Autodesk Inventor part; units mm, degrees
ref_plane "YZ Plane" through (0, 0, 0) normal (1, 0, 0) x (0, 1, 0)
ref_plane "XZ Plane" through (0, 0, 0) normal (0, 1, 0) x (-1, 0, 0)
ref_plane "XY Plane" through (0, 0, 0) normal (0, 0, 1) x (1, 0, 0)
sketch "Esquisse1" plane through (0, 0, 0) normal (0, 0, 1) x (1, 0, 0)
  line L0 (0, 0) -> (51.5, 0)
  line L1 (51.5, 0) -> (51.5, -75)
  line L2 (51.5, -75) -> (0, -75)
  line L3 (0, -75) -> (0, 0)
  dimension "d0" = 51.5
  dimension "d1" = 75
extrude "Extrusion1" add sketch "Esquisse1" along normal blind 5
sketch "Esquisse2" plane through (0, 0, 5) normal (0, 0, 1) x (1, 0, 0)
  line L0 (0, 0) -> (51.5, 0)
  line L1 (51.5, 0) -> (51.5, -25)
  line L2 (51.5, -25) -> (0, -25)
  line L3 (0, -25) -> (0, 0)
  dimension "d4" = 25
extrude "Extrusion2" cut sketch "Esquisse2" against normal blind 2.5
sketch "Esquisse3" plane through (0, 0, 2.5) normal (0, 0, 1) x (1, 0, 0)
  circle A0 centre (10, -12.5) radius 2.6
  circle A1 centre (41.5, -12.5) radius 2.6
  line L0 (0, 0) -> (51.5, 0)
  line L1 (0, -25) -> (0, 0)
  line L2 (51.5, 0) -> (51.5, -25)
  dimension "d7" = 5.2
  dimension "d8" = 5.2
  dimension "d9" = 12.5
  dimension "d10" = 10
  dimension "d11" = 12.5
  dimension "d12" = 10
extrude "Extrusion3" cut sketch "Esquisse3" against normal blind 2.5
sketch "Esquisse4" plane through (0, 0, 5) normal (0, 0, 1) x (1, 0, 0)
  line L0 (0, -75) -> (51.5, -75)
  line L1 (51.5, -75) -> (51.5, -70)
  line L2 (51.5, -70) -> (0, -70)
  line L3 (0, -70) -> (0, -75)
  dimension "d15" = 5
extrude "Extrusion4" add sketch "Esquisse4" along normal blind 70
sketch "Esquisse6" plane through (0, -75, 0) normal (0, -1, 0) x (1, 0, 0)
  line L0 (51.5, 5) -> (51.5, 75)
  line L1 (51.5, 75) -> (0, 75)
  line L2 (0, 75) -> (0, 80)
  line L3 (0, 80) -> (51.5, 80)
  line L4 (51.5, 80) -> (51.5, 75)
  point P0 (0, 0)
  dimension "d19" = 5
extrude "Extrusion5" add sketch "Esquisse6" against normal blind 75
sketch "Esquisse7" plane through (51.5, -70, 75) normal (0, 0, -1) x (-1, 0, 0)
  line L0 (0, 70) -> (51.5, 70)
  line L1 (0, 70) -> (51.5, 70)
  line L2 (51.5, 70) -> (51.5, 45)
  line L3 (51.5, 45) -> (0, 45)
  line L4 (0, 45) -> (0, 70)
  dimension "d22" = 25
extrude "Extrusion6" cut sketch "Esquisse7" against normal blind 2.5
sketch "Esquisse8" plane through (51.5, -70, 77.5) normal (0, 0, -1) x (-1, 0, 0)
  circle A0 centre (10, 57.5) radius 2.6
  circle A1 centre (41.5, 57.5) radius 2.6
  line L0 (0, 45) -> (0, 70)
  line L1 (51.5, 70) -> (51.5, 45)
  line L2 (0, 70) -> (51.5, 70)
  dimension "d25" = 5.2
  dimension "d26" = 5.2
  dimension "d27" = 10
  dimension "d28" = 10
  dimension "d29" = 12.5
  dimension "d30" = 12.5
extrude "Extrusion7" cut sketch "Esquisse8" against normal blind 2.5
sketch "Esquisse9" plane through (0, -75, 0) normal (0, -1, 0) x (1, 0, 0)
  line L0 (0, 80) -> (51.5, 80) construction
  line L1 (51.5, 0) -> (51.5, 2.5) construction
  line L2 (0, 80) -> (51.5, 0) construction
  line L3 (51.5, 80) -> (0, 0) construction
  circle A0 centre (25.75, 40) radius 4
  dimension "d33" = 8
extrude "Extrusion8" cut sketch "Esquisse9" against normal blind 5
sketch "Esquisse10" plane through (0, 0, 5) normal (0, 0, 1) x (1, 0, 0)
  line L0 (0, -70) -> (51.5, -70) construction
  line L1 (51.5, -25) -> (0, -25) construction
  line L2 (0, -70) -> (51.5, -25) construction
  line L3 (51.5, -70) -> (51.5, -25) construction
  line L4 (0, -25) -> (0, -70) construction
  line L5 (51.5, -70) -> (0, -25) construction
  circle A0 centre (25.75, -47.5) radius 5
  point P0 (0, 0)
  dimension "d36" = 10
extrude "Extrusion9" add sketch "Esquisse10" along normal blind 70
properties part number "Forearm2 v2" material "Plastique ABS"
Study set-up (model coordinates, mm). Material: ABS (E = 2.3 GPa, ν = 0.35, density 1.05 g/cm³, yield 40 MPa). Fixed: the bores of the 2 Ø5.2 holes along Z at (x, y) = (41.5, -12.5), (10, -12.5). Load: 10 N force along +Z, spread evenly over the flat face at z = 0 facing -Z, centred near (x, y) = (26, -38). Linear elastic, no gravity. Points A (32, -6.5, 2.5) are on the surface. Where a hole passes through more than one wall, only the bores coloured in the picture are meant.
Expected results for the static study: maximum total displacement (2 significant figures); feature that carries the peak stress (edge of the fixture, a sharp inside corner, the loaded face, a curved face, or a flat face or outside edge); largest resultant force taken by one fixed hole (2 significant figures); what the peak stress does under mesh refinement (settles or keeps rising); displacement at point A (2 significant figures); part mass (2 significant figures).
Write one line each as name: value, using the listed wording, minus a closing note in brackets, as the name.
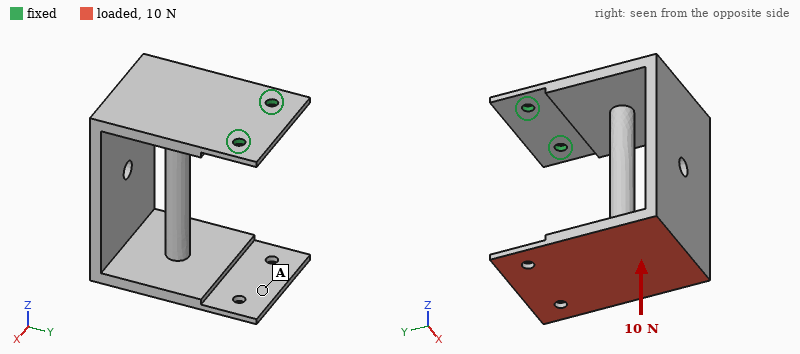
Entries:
maximum total displacement: 1.4 mm
feature that carries the peak stress: edge of the fixture
largest resultant force taken by one fixed hole: 5.0 N
what the peak stress does under mesh refinement: keeps rising
displacement at point A: 1.1 mm
part mass: 58 g
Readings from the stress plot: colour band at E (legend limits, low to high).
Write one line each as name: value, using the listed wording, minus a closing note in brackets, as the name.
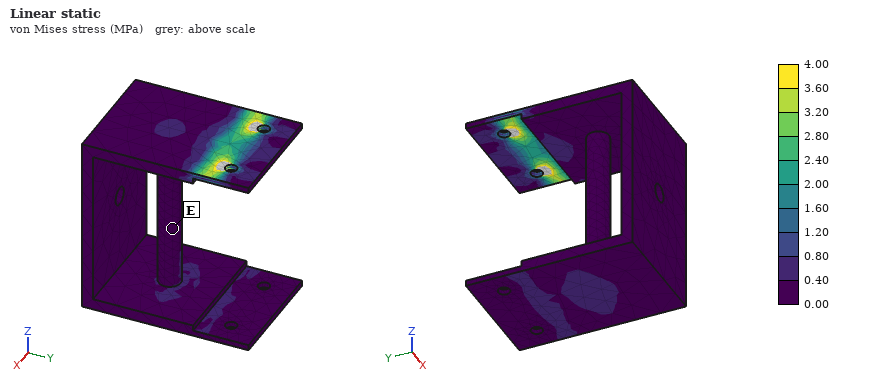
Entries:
colour band at E: 0.00 to 0.40 MPa
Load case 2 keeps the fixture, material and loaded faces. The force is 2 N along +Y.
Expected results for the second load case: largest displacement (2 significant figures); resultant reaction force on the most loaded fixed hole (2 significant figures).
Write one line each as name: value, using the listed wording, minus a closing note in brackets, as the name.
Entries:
largest displacement: 1.4 mm
resultant reaction force on the most loaded fixed hole: 1.0 N
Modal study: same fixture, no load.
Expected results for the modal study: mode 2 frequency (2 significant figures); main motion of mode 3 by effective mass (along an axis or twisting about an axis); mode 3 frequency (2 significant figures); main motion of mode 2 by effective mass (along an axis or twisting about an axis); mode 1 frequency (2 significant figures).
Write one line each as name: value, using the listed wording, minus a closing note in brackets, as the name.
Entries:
mode 2 frequency: 76 Hz
main motion of mode 3 by effective mass: along Z
mode 3 frequency: 240 Hz
main motion of mode 2 by effective mass: along X
mode 1 frequency: 34 Hz
